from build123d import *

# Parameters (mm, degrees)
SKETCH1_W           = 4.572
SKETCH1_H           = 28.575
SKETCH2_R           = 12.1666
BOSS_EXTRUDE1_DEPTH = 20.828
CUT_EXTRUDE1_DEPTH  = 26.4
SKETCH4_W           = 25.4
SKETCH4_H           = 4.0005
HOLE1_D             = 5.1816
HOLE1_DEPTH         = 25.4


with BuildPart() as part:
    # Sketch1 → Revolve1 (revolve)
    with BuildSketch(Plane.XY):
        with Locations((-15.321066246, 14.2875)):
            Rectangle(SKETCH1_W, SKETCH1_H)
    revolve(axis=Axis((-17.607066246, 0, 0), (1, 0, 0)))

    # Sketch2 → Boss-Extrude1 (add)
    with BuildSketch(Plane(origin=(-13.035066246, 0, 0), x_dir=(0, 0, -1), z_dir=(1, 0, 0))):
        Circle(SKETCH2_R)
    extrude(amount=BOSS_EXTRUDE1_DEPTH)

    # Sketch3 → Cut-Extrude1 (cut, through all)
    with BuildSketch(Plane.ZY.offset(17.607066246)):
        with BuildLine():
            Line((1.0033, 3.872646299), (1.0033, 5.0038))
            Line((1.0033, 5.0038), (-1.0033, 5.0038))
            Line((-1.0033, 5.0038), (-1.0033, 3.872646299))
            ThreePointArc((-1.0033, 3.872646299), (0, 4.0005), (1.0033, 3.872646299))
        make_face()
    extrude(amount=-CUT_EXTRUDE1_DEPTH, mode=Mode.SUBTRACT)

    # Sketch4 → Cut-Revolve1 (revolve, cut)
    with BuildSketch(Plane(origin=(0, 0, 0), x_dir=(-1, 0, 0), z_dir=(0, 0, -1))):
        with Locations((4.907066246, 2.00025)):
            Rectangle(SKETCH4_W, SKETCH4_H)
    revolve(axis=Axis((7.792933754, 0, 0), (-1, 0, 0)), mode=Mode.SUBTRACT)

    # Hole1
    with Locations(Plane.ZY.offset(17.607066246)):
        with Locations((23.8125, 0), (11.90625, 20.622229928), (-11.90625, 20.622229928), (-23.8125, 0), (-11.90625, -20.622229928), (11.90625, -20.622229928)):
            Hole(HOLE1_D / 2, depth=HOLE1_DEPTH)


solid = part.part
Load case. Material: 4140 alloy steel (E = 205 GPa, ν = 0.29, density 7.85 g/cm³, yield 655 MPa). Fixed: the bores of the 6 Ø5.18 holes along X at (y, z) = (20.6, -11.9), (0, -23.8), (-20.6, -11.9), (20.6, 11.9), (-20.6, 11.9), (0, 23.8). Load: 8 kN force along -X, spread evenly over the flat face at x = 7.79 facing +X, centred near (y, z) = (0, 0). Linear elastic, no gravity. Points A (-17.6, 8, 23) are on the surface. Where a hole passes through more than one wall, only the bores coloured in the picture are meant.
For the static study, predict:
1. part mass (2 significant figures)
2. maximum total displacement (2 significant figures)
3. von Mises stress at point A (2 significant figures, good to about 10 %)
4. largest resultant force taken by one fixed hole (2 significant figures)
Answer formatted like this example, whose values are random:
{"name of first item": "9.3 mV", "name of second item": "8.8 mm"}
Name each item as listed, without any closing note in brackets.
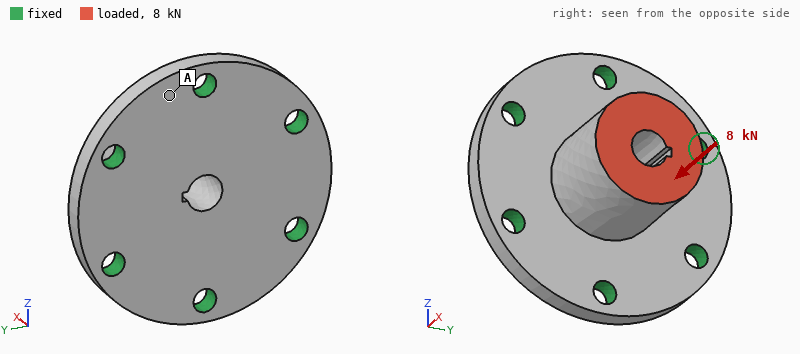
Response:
{"part mass": "150 g", "maximum total displacement": "15 µm", "von Mises stress at point A": "32 MPa", "largest resultant force taken by one fixed hole": "1.4 kN"}
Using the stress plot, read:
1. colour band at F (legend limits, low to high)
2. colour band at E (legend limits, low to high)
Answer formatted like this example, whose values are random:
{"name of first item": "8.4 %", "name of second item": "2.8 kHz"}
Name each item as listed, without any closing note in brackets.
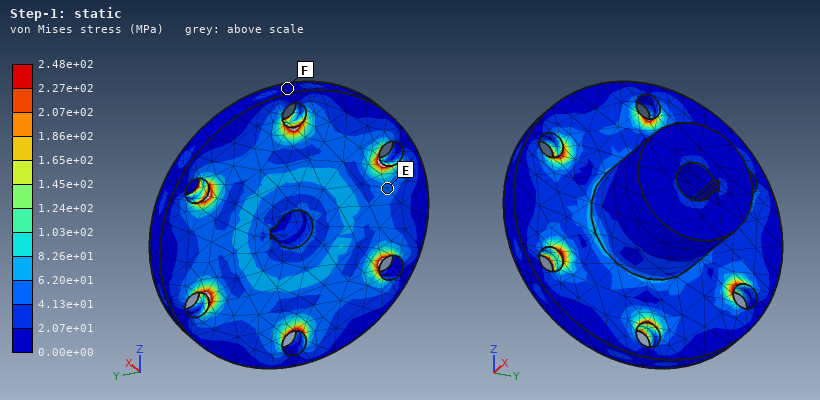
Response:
{"colour band at F": "0.00e+00 to 2.07e+01 MPa", "colour band at E": "4.13e+01 to 6.20e+01 MPa"}
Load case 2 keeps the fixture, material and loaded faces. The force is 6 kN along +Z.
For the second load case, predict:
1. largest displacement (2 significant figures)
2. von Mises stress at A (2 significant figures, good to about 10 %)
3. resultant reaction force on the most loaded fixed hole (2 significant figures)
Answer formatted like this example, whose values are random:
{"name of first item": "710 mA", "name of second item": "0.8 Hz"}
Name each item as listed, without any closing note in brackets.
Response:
{"largest displacement": "48 µm", "von Mises stress at A": "44 MPa", "resultant reaction force on the most loaded fixed hole": "3.0 kN"}
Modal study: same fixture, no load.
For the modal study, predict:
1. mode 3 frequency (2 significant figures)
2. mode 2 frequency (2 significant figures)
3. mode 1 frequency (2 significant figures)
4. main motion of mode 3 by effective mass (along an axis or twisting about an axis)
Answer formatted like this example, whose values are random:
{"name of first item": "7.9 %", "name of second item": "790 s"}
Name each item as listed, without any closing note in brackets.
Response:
{"mode 3 frequency": "13 kHz", "mode 2 frequency": "11 kHz", "mode 1 frequency": "11 kHz", "main motion of mode 3 by effective mass": "along X"}
